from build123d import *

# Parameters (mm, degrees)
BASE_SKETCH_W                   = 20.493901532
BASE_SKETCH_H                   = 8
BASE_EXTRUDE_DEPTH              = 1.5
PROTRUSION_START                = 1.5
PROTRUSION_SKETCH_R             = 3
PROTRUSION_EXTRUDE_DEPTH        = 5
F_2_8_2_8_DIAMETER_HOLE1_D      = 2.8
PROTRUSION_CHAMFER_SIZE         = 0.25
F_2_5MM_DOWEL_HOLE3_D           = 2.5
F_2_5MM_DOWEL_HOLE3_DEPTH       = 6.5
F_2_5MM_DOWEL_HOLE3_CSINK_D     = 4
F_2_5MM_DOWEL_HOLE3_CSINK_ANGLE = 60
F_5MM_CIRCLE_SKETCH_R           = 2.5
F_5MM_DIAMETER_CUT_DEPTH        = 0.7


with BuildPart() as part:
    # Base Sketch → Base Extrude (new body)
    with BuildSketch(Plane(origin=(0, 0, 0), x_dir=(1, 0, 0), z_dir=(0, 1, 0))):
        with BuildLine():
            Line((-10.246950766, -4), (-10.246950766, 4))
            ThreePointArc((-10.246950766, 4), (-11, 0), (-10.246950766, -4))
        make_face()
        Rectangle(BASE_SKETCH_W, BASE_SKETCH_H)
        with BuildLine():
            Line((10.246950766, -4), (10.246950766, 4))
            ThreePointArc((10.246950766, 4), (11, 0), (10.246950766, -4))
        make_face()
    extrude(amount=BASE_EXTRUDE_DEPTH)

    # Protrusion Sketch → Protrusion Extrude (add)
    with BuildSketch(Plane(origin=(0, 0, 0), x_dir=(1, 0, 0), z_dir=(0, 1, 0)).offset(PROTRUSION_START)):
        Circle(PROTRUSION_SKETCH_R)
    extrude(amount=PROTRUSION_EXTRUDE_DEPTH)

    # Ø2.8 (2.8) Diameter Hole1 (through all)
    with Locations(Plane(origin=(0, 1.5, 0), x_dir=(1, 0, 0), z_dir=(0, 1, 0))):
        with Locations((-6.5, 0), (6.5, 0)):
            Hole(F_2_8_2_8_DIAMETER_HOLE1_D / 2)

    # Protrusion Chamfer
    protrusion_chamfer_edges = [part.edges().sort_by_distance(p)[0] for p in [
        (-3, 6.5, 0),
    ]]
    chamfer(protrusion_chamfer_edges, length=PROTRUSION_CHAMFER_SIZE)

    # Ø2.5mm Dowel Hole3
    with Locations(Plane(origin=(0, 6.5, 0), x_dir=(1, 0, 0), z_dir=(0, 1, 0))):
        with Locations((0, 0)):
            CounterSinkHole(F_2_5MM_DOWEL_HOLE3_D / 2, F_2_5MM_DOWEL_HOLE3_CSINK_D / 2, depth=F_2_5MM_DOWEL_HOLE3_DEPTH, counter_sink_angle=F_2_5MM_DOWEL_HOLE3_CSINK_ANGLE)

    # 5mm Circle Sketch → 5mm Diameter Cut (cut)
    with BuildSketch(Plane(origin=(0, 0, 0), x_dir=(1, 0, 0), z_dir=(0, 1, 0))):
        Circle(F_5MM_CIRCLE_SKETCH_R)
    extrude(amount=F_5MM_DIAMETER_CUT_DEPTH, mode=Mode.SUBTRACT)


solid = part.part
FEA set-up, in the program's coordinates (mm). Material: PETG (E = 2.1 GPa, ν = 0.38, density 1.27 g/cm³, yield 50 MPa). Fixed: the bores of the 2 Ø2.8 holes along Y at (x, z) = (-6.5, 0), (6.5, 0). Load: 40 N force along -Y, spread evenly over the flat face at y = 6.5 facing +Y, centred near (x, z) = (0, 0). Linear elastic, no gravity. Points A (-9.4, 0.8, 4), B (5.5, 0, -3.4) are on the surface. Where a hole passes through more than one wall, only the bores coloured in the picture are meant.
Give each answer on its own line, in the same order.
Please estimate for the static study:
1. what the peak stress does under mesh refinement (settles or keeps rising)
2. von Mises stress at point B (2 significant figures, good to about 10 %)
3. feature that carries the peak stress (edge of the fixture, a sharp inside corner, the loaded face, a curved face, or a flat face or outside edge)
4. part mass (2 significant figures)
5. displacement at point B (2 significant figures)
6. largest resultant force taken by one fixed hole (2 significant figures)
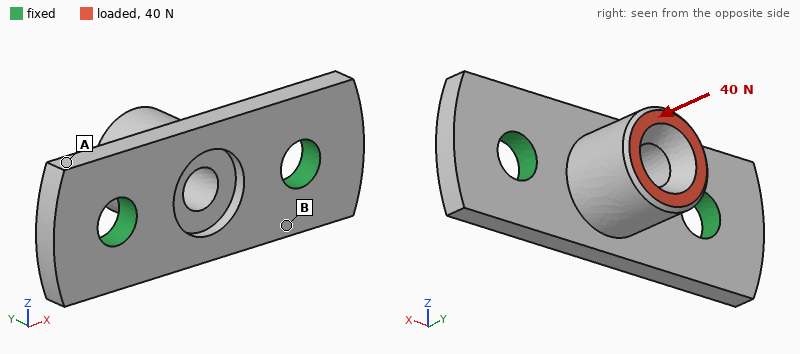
keeps rising
3.8 MPa
edge of the fixture
0.42 g
7.0 µm
23 N
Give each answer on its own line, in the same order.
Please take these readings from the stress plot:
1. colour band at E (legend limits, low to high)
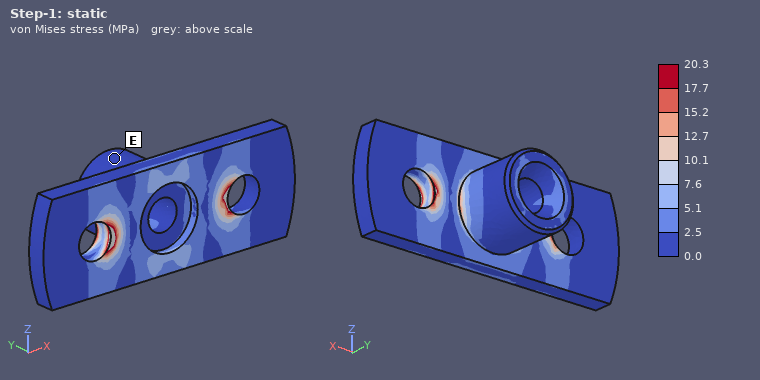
0.0 to 2.5 MPa
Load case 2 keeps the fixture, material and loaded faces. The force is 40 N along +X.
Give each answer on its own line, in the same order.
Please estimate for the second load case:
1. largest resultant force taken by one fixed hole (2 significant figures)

34 N
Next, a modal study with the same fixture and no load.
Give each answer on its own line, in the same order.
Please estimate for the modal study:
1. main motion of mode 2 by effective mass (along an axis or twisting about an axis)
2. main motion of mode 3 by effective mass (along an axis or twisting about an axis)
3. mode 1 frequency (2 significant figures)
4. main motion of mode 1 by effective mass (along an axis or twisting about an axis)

along Y
along X
6400 Hz
along Z
